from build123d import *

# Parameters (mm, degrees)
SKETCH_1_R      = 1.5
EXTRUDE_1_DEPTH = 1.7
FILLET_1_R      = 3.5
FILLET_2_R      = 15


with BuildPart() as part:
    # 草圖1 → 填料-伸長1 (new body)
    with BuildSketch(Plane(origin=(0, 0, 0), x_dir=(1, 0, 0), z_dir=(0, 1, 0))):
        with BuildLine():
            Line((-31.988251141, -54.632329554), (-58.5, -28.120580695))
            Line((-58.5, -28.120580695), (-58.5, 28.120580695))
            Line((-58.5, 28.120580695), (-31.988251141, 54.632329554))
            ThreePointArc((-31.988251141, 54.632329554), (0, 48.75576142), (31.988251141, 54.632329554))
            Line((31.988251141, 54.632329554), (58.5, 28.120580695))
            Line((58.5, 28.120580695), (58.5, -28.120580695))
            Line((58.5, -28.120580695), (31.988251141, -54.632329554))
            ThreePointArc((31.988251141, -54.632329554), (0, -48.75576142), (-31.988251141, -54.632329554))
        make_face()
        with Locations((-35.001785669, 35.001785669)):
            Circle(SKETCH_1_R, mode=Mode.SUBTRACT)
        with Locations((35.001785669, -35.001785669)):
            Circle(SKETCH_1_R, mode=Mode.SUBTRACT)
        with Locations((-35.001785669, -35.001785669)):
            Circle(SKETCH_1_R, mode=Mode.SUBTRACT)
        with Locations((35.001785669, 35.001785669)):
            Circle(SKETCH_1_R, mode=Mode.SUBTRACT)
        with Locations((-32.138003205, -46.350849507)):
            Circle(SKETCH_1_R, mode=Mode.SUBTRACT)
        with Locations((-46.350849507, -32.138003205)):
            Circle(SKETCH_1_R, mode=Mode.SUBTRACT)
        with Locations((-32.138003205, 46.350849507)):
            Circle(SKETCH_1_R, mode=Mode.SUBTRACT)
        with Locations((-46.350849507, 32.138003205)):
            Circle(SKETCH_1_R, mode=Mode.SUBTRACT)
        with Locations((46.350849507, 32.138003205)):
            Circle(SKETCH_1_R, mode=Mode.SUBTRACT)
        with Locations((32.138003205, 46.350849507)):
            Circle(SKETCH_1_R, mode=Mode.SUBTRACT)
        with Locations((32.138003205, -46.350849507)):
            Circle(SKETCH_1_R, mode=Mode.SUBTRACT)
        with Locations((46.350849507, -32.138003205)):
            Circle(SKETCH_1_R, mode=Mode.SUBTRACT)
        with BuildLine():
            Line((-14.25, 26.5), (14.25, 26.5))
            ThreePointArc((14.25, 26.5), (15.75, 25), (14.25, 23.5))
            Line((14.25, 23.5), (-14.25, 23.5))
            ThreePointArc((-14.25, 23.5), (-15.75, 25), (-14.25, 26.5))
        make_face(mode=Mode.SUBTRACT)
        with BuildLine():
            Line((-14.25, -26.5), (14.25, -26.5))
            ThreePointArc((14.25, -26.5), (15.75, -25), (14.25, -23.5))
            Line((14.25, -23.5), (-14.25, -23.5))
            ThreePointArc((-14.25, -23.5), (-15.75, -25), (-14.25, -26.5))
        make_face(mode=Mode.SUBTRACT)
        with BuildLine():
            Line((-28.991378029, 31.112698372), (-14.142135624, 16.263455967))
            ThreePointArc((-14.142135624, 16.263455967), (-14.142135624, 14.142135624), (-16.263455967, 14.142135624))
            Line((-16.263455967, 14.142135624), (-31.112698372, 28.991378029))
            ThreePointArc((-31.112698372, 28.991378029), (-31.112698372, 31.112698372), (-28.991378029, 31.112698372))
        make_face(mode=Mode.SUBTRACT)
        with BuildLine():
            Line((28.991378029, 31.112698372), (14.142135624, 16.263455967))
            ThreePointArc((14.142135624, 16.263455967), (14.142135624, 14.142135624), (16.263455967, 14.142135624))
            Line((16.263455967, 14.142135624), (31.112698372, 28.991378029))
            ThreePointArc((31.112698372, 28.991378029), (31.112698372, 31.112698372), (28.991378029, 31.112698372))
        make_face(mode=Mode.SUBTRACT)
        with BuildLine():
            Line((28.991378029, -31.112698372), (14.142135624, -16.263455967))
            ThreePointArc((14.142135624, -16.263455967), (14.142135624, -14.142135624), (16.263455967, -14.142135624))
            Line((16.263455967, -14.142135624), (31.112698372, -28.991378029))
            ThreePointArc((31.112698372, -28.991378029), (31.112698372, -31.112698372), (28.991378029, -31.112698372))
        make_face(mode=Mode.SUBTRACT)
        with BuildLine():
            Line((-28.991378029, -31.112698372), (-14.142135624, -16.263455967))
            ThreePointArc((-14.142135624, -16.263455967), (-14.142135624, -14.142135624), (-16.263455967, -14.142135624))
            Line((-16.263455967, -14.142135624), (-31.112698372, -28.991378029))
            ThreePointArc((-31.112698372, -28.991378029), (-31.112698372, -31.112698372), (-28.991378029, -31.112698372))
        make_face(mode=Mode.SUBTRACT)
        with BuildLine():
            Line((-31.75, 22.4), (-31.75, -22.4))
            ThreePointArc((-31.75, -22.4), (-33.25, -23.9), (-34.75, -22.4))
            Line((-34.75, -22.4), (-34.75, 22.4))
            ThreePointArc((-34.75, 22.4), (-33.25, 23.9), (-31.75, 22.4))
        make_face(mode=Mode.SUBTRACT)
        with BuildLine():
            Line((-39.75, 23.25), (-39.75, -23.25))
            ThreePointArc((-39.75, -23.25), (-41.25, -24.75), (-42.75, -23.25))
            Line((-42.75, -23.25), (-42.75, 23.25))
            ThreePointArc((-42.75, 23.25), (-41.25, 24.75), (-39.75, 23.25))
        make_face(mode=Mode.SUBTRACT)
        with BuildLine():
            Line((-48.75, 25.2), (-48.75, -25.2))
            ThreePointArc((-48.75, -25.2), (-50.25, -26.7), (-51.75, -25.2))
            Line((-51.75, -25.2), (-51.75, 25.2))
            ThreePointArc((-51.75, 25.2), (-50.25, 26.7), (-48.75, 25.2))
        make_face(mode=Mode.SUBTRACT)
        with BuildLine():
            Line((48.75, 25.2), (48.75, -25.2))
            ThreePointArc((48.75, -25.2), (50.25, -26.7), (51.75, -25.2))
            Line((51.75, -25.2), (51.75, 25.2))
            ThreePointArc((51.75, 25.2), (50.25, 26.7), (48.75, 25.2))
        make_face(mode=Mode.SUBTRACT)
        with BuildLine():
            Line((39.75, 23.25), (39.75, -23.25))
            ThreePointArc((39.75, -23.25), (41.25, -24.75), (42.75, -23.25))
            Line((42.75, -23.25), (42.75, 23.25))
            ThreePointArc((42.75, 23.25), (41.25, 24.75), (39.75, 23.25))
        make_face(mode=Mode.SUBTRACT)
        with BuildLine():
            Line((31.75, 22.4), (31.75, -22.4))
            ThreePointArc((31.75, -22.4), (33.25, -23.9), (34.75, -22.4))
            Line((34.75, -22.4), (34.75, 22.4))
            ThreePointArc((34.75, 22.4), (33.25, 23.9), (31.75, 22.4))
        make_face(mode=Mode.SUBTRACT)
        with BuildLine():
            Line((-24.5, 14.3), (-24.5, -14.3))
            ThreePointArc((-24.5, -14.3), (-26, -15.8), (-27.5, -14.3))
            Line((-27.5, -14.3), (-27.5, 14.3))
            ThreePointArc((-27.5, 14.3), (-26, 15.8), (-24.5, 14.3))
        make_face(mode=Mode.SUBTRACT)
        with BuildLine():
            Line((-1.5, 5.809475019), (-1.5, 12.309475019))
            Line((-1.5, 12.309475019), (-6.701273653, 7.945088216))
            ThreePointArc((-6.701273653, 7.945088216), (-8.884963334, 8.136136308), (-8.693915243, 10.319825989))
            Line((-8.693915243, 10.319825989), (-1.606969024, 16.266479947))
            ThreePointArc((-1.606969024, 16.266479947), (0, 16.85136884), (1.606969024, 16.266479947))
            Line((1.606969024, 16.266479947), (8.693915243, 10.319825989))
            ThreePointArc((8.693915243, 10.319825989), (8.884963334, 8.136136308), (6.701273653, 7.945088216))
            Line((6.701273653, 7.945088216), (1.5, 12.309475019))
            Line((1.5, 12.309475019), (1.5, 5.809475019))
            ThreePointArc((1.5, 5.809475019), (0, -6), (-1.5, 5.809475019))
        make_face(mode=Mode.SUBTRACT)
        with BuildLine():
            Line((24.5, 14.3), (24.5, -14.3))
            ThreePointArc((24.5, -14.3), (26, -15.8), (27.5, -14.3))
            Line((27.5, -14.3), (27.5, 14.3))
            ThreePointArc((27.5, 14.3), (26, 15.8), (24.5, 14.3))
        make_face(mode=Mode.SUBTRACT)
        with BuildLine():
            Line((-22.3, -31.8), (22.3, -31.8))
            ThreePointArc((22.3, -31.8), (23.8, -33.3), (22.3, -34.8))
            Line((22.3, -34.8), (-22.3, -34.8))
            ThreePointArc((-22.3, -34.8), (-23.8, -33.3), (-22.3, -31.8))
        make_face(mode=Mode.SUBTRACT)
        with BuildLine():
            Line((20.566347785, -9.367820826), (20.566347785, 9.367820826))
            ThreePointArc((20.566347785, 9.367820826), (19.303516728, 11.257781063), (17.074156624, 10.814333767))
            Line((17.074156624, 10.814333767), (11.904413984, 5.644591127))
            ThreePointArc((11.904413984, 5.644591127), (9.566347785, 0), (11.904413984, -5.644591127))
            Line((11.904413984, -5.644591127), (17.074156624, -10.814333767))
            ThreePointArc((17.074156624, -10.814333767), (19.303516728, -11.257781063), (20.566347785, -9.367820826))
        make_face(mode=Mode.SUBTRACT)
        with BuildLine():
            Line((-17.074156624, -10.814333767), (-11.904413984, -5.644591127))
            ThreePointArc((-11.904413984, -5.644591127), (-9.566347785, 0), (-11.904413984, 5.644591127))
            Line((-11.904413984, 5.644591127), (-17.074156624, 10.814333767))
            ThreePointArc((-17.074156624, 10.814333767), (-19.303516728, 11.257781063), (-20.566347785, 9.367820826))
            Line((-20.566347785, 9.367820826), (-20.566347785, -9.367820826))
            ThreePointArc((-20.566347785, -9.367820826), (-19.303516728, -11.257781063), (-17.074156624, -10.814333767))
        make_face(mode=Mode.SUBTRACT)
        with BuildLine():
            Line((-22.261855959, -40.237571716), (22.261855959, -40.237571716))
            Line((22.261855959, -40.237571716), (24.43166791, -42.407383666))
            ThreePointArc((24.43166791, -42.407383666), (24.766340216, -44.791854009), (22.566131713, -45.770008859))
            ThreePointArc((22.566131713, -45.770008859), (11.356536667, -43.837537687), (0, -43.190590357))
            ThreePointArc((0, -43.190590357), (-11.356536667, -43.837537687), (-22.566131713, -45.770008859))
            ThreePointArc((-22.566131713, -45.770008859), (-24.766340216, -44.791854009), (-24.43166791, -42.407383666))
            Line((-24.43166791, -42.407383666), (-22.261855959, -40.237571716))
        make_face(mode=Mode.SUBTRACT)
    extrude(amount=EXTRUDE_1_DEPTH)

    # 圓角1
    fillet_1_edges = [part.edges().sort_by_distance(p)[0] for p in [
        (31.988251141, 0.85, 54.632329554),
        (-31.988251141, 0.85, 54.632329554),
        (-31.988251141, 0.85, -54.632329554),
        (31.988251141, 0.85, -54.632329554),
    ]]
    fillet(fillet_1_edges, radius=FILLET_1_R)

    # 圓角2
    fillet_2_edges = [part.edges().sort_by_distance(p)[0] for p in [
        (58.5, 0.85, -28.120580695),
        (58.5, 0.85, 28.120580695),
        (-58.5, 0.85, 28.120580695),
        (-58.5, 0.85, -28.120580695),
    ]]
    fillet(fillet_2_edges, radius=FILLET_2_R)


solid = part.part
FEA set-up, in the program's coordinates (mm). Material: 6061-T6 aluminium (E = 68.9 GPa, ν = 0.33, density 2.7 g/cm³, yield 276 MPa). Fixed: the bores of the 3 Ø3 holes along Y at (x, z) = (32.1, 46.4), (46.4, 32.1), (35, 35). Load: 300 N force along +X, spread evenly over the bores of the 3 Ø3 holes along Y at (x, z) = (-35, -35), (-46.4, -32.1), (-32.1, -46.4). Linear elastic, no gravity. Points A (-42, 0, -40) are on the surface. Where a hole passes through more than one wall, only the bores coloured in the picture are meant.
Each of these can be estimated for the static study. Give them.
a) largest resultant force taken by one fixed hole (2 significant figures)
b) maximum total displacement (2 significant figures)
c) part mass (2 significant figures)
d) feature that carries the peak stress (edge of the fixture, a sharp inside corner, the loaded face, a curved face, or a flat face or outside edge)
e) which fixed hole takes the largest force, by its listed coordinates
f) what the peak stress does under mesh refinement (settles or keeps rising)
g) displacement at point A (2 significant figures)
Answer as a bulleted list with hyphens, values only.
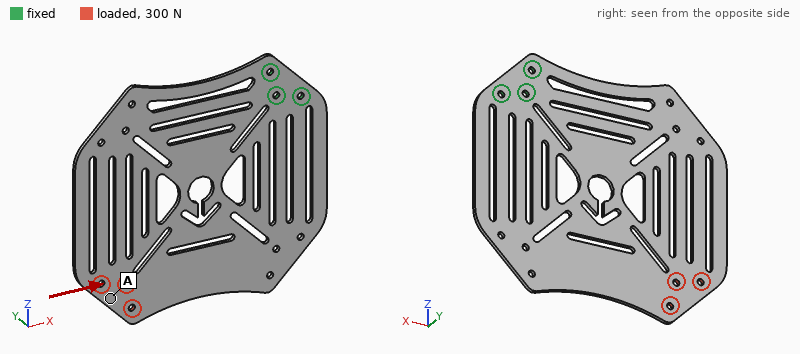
- 960 N
- 0.55 mm
- 38 g
- a sharp inside corner
- (46.4, 32.1)
- keeps rising
- 0.53 mm
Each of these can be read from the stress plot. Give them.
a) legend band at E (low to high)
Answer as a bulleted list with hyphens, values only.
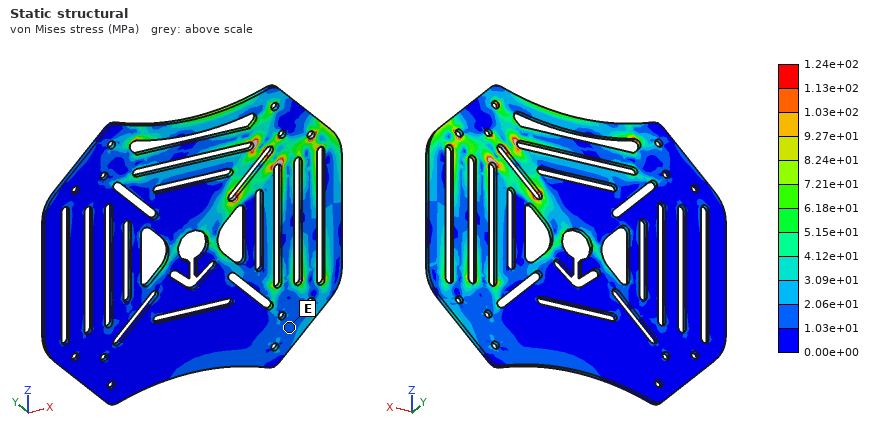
- 1.03e+01 to 2.06e+01 MPa
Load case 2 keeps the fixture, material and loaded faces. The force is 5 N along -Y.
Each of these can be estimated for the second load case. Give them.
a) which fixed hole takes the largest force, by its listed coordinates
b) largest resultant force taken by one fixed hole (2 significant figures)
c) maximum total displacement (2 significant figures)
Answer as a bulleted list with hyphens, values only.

- (35, 35)
- 22 N
- 1.9 mm
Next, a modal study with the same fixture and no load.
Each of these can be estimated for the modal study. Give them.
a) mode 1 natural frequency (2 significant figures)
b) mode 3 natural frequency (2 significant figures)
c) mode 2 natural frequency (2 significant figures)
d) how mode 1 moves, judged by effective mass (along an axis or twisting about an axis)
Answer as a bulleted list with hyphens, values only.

- 87 Hz
- 410 Hz
- 190 Hz
- along Y
